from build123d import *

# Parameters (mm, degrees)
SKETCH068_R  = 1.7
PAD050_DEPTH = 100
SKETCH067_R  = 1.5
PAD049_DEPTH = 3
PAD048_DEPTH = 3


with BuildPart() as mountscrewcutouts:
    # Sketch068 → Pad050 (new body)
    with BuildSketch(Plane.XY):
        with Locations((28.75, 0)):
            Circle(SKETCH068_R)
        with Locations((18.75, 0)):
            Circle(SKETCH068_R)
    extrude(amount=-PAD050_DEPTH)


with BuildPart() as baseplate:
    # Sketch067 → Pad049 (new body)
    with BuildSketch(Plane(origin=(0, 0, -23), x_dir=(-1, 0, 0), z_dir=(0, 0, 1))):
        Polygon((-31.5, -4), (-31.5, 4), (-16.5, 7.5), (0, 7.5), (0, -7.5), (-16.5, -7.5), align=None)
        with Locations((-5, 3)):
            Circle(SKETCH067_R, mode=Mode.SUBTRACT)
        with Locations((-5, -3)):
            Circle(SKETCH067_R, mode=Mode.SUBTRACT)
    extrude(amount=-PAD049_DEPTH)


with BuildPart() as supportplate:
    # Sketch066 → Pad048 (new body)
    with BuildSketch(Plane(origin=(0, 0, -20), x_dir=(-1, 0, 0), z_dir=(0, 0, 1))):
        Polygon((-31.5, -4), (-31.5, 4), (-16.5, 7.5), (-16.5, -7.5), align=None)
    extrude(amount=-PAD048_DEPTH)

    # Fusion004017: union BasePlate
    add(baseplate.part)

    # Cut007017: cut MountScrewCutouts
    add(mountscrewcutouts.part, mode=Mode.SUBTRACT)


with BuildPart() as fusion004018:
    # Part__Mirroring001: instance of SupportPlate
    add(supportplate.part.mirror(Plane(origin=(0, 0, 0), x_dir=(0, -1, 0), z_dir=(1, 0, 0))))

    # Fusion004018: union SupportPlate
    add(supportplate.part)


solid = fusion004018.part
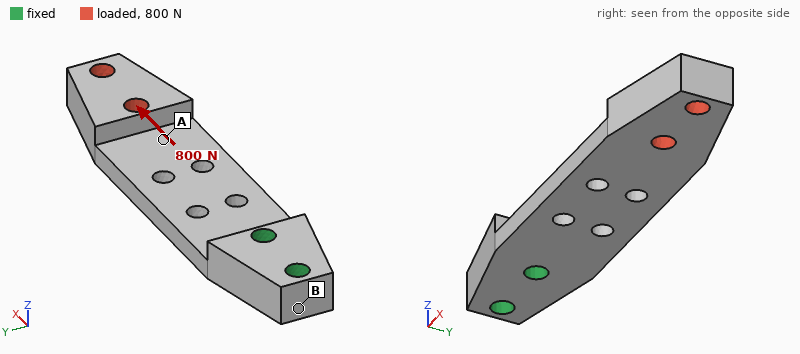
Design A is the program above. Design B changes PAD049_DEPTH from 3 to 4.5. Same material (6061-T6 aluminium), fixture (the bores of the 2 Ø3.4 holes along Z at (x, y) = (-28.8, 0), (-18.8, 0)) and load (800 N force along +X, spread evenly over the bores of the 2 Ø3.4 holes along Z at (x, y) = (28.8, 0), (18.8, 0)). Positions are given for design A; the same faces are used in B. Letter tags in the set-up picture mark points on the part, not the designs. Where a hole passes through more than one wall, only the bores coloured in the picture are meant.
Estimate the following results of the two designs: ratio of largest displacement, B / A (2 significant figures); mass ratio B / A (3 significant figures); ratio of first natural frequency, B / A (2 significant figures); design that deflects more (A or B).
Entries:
0.31
1.36
1.6
A
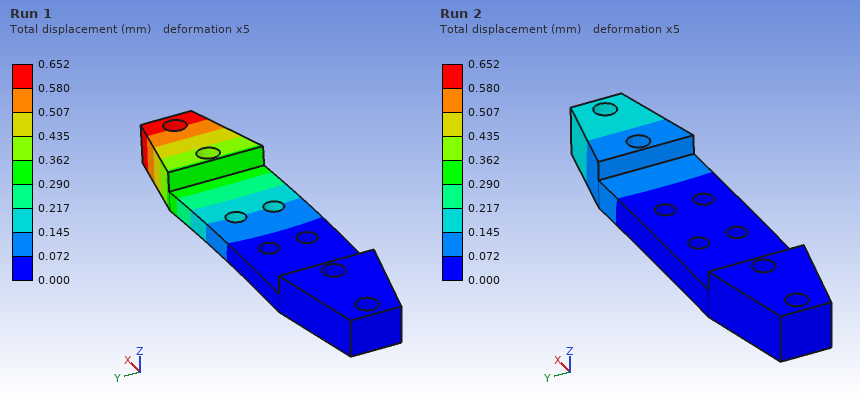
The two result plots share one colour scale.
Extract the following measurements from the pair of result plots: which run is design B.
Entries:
Run 2
